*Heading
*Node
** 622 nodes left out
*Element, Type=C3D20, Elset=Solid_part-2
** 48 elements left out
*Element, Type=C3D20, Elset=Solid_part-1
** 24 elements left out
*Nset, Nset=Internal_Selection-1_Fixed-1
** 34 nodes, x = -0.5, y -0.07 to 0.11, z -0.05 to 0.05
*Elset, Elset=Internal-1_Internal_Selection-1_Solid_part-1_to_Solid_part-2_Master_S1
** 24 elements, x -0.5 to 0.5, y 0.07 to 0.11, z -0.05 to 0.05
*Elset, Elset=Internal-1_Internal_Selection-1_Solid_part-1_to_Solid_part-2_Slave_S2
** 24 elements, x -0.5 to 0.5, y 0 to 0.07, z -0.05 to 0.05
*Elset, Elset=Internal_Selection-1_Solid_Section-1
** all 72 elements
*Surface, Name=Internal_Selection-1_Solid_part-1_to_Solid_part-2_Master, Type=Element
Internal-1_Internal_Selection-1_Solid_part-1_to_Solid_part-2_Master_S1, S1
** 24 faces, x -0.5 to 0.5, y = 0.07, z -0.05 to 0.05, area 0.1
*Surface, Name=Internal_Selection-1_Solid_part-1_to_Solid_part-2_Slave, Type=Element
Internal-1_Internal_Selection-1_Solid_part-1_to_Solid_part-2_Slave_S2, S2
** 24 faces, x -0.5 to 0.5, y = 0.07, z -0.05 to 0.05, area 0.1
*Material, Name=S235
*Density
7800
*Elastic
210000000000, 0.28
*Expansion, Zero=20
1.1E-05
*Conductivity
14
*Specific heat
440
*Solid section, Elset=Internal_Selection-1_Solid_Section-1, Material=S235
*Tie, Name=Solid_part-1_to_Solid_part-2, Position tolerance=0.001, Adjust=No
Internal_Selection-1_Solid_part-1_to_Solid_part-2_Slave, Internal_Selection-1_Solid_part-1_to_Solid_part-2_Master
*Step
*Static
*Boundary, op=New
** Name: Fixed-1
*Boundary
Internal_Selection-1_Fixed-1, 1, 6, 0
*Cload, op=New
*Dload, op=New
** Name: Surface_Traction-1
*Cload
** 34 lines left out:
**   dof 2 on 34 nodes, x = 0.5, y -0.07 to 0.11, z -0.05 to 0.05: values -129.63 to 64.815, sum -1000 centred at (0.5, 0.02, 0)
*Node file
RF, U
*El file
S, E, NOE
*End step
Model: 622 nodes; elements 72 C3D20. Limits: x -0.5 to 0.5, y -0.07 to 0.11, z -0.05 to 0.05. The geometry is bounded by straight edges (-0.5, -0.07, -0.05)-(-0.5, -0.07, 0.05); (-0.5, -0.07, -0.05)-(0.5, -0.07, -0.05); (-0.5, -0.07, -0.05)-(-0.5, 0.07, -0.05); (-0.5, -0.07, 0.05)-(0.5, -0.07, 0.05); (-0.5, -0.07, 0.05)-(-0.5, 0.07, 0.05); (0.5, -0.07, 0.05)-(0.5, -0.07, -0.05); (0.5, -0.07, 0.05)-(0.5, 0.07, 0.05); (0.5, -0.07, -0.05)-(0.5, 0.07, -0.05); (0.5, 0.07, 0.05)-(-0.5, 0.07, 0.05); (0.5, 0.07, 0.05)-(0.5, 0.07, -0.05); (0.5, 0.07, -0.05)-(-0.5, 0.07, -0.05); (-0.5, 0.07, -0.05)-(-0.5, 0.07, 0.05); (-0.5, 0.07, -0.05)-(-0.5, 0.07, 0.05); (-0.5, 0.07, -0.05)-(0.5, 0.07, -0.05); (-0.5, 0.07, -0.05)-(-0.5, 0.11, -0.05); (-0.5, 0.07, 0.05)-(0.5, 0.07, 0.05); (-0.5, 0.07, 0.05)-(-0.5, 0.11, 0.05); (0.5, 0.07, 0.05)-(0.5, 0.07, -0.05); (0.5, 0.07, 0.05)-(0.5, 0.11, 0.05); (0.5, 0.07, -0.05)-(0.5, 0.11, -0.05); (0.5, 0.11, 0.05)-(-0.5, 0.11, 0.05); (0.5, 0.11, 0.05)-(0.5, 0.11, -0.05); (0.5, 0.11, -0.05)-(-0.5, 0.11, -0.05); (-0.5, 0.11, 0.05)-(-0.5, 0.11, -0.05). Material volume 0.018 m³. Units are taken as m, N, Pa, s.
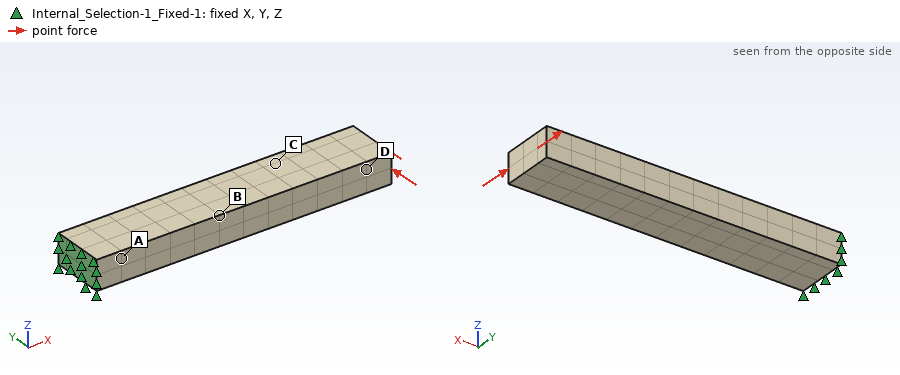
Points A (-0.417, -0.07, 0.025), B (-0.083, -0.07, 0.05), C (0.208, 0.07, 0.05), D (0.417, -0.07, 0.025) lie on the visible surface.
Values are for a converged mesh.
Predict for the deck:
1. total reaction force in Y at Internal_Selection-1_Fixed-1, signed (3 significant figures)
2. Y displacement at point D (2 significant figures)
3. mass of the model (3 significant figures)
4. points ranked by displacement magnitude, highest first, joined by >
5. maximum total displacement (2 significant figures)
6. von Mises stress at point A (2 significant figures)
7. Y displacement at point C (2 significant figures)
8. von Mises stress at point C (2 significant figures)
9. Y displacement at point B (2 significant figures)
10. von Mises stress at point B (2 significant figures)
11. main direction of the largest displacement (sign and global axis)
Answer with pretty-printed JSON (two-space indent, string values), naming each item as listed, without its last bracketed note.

{
  "total reaction force in Y at Internal_Selection-1_Fixed-1, signed": "1000 N",
  "Y displacement at point D": "-2.9e-05 m",
  "mass of the model": "140 kg",
  "points ranked by displacement magnitude, highest first, joined by >": "D > C > B > A",
  "maximum total displacement": "3.4e-05 m",
  "von Mises stress at point A": "1.7e+06 Pa",
  "Y displacement at point C": "-1.9e-05 m",
  "von Mises stress at point C": "3.2e+05 Pa",
  "Y displacement at point B": "-7.6e-06 m",
  "von Mises stress at point B": "1.1e+06 Pa",
  "main direction of the largest displacement": "-Y"
}
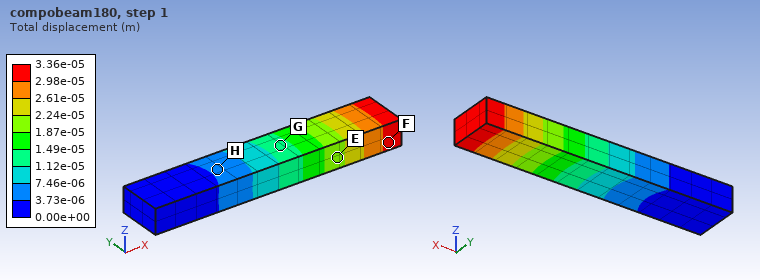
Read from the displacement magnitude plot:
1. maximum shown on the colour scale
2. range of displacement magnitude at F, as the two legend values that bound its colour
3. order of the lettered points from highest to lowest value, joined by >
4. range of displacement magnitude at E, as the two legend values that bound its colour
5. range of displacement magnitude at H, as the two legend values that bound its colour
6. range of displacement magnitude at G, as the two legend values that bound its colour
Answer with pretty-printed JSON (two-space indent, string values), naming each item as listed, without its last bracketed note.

{
  "maximum shown on the colour scale": "3.36e-05 m",
  "range of displacement magnitude at F, as the two legend values that bound its colour": "2.98e-05 to 3.36e-05 m",
  "order of the lettered points from highest to lowest value, joined by >": "F > E > G > H",
  "range of displacement magnitude at E, as the two legend values that bound its colour": "1.87e-05 to 2.24e-05 m",
  "range of displacement magnitude at H, as the two legend values that bound its colour": "3.73e-06 to 7.46e-06 m",
  "range of displacement magnitude at G, as the two legend values that bound its colour": "1.12e-05 to 1.49e-05 m"
}
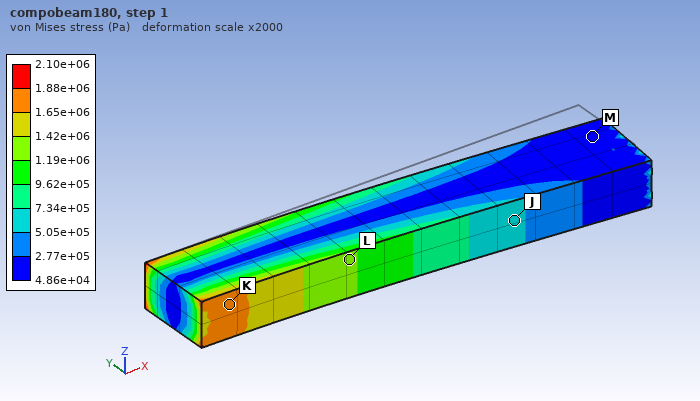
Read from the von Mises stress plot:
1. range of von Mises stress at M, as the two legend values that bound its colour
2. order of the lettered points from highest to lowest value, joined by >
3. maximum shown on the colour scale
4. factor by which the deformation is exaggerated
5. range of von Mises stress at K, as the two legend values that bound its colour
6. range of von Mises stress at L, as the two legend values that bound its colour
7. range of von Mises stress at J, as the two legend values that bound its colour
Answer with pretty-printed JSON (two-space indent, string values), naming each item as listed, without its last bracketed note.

{
  "range of von Mises stress at M, as the two legend values that bound its colour": "4.86e+04 to 2.77e+05 Pa",
  "order of the lettered points from highest to lowest value, joined by >": "K > L > J > M",
  "maximum shown on the colour scale": "2.10e+06 Pa",
  "factor by which the deformation is exaggerated": "2000",
  "range of von Mises stress at K, as the two legend values that bound its colour": "1.65e+06 to 1.88e+06 Pa",
  "range of von Mises stress at L, as the two legend values that bound its colour": "1.19e+06 to 1.42e+06 Pa",
  "range of von Mises stress at J, as the two legend values that bound its colour": "5.05e+05 to 7.34e+05 Pa"
}
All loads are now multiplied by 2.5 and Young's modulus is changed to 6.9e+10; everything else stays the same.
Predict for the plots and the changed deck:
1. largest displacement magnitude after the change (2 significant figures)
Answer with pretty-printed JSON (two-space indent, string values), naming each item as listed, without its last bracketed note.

{
  "largest displacement magnitude after the change": "2.6e-04 m"
}
